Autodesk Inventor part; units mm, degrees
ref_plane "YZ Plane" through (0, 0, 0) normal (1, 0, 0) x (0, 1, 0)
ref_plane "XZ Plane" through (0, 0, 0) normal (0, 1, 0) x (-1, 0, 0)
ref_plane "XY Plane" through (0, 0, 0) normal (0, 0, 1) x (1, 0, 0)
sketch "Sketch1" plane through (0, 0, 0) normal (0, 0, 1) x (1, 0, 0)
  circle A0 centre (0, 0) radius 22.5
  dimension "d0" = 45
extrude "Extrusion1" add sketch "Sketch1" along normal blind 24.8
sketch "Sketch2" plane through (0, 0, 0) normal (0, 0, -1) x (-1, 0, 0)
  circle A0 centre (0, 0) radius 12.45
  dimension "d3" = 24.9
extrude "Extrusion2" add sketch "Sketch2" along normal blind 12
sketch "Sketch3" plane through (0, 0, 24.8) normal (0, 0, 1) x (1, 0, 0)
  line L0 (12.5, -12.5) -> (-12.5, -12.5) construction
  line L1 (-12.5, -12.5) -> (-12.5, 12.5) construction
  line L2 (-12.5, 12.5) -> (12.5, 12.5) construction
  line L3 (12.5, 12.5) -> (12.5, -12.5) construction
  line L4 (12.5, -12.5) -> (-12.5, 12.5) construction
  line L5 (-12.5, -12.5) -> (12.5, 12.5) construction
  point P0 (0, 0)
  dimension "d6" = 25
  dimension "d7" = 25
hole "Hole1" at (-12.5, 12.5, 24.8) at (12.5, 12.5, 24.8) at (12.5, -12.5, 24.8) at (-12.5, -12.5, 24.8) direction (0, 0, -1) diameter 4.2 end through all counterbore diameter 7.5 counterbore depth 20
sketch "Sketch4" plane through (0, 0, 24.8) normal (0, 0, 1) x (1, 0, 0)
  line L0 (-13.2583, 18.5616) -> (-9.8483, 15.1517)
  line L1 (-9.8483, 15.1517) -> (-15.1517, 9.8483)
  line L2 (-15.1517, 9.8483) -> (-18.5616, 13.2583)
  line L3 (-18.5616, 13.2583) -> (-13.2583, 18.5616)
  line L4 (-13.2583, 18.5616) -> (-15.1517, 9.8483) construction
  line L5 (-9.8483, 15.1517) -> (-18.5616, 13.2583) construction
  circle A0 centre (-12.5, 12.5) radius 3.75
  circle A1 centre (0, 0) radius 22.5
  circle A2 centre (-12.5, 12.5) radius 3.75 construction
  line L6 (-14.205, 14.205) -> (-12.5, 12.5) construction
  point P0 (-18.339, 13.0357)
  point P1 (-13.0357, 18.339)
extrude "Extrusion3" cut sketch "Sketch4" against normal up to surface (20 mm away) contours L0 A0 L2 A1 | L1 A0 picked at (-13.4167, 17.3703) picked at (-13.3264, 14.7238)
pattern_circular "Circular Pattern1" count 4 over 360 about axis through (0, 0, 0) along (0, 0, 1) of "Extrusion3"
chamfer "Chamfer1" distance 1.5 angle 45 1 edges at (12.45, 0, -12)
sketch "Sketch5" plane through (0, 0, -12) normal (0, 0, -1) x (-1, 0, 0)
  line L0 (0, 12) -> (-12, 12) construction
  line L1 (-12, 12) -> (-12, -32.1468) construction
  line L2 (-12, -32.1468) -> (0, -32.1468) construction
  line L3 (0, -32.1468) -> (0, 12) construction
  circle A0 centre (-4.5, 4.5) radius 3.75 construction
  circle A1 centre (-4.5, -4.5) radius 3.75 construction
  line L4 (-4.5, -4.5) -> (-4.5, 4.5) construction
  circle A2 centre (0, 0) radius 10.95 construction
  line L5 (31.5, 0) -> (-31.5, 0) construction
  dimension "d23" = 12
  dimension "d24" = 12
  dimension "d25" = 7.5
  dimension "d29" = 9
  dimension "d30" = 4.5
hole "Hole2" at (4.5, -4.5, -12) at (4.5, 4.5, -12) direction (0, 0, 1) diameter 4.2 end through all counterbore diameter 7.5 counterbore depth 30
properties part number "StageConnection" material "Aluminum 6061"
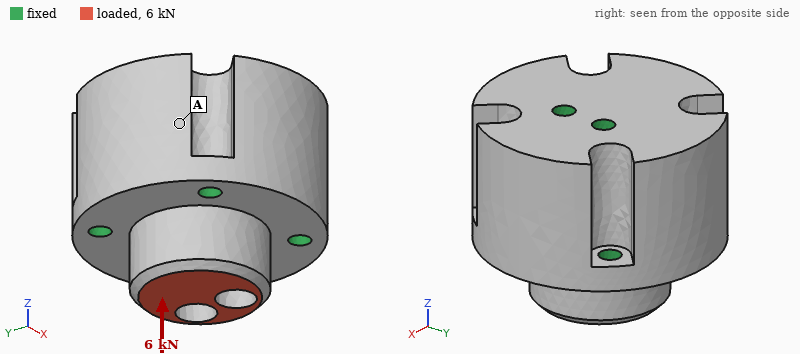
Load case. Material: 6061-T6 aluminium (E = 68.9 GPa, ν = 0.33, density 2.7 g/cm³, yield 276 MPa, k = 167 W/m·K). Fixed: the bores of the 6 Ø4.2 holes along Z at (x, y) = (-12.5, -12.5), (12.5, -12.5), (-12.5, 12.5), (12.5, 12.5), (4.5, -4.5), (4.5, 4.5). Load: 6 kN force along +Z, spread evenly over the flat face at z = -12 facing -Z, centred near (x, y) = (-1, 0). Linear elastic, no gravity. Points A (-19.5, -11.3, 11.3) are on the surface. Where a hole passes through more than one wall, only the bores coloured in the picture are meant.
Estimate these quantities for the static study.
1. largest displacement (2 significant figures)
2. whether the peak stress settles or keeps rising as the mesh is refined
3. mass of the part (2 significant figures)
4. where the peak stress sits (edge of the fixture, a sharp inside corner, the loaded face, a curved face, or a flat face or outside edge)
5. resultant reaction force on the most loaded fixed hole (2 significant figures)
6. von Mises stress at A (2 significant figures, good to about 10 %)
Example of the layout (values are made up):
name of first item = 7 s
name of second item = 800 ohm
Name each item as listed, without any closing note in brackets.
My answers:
largest displacement = 7.2 µm
whether the peak stress settles or keeps rising as the mesh is refined = keeps rising
mass of the part = 100 g
where the peak stress sits = edge of the fixture
resultant reaction force on the most loaded fixed hole = 1.2 kN
von Mises stress at A = 5.9 MPa
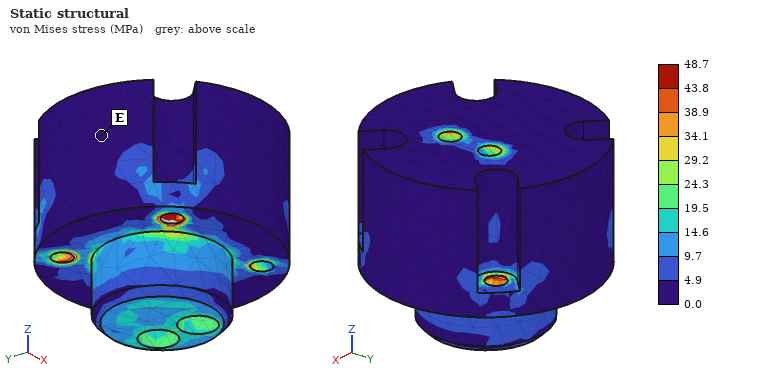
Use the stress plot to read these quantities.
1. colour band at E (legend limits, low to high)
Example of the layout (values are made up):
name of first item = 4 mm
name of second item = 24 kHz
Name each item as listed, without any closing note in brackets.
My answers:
colour band at E = 0.0 to 4.9 MPa
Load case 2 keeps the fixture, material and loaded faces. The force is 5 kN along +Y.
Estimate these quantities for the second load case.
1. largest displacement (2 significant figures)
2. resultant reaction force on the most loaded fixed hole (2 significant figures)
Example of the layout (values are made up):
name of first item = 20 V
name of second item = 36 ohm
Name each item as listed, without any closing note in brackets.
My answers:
largest displacement = 23 µm
resultant reaction force on the most loaded fixed hole = 2.0 kN
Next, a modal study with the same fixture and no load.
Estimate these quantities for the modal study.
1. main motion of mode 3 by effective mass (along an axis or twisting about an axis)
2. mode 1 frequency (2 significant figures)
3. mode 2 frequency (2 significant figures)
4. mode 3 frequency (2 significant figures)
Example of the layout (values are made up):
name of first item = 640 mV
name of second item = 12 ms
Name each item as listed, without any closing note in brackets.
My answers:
main motion of mode 3 by effective mass = along Y
mode 1 frequency = 24 kHz
mode 2 frequency = 24 kHz
mode 3 frequency = 27 kHz
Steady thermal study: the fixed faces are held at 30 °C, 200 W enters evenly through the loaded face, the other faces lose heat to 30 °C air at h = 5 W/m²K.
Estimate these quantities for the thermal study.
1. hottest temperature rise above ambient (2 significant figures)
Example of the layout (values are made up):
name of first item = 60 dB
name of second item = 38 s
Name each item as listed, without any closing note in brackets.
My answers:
hottest temperature rise above ambient = 66 K
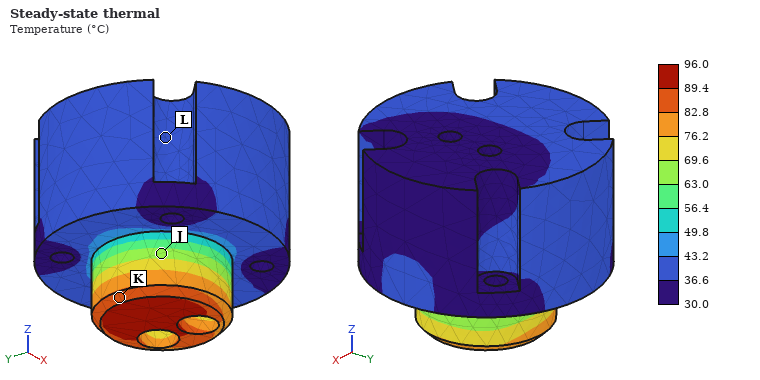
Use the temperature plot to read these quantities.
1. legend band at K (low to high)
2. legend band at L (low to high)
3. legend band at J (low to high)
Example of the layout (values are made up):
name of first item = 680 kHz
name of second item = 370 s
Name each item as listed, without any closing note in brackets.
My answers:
legend band at K = 82.8 to 89.4 °C
legend band at L = 36.6 to 43.2 °C
legend band at J = 63.0 to 69.6 °C
